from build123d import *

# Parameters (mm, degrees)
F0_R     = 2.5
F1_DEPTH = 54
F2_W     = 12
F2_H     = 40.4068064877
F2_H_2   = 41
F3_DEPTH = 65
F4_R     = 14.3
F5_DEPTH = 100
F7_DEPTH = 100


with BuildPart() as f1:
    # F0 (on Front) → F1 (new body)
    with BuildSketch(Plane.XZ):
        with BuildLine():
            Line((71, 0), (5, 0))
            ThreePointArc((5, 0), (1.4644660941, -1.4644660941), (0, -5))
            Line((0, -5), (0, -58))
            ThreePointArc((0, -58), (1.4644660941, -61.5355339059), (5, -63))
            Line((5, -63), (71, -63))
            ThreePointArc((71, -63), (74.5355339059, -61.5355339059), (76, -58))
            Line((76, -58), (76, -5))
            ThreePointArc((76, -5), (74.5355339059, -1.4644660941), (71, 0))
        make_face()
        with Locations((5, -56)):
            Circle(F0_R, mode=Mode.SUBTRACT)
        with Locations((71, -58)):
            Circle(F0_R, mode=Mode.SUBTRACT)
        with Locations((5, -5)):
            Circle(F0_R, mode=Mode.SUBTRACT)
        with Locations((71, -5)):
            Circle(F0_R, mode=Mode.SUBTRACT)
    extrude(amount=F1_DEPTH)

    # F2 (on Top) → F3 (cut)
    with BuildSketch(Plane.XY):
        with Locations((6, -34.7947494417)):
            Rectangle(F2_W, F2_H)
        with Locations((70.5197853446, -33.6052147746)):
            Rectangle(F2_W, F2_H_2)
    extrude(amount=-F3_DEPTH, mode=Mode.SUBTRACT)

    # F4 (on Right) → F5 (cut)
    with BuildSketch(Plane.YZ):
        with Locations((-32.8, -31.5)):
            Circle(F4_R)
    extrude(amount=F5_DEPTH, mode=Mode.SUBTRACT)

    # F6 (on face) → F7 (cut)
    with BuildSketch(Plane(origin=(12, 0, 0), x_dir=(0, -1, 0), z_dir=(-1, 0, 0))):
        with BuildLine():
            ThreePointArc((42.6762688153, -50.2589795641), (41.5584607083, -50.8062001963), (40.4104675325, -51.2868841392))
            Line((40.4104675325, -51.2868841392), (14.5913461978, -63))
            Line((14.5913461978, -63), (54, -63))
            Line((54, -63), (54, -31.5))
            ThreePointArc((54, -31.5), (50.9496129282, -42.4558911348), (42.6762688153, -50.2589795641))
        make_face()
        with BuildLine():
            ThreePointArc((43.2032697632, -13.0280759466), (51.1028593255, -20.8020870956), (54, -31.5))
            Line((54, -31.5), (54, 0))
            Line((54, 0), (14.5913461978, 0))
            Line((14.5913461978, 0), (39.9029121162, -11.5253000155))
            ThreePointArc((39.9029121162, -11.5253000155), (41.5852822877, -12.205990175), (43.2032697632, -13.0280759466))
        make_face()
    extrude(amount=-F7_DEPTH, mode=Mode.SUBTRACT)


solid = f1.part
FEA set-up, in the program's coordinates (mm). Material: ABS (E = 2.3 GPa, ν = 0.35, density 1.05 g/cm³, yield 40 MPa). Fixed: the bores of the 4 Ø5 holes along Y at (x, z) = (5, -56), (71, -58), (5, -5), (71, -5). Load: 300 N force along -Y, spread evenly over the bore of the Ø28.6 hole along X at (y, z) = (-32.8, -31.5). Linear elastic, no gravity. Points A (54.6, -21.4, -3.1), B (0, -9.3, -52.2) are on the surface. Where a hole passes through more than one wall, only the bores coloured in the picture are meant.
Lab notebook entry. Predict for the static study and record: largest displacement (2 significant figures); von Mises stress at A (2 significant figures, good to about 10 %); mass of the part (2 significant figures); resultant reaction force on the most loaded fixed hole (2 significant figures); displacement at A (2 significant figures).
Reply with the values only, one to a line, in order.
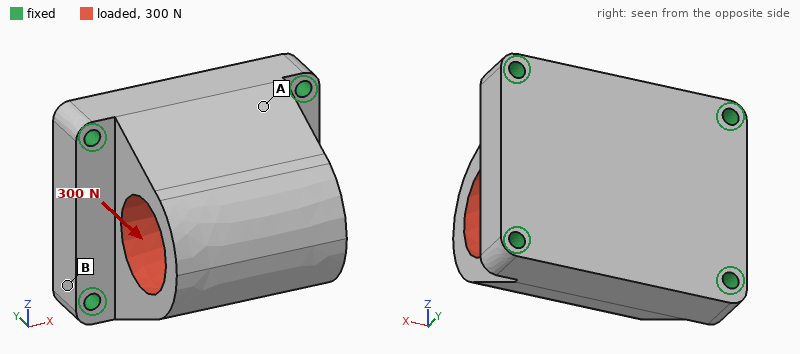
12 µm
0.29 MPa
130 g
82 N
7.1 µm
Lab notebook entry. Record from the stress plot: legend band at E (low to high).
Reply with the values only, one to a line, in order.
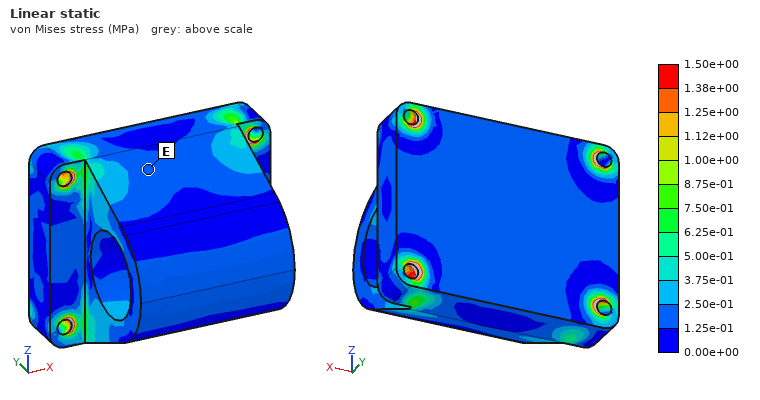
1.25e-01 to 2.50e-01 MPa
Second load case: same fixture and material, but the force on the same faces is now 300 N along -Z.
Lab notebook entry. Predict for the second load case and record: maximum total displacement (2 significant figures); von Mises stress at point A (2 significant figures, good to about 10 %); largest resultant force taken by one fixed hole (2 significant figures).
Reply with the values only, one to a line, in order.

32 µm
0.46 MPa
120 N
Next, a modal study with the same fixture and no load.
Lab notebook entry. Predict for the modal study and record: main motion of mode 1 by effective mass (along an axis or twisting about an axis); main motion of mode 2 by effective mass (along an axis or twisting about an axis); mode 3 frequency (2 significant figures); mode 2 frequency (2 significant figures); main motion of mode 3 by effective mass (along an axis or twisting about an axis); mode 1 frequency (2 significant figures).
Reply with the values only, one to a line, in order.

along Z
along Y
3100 Hz
2900 Hz
along X
2400 Hz
